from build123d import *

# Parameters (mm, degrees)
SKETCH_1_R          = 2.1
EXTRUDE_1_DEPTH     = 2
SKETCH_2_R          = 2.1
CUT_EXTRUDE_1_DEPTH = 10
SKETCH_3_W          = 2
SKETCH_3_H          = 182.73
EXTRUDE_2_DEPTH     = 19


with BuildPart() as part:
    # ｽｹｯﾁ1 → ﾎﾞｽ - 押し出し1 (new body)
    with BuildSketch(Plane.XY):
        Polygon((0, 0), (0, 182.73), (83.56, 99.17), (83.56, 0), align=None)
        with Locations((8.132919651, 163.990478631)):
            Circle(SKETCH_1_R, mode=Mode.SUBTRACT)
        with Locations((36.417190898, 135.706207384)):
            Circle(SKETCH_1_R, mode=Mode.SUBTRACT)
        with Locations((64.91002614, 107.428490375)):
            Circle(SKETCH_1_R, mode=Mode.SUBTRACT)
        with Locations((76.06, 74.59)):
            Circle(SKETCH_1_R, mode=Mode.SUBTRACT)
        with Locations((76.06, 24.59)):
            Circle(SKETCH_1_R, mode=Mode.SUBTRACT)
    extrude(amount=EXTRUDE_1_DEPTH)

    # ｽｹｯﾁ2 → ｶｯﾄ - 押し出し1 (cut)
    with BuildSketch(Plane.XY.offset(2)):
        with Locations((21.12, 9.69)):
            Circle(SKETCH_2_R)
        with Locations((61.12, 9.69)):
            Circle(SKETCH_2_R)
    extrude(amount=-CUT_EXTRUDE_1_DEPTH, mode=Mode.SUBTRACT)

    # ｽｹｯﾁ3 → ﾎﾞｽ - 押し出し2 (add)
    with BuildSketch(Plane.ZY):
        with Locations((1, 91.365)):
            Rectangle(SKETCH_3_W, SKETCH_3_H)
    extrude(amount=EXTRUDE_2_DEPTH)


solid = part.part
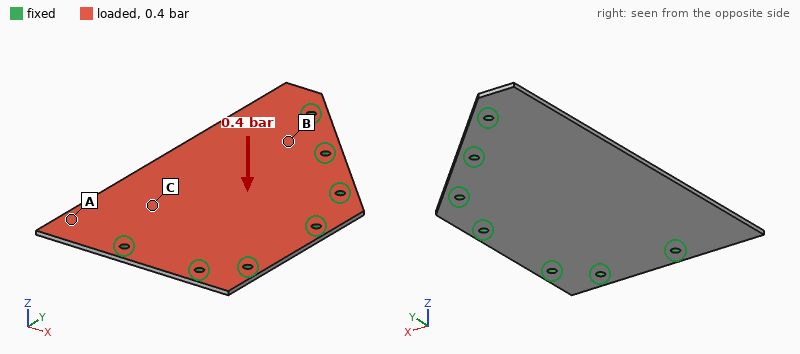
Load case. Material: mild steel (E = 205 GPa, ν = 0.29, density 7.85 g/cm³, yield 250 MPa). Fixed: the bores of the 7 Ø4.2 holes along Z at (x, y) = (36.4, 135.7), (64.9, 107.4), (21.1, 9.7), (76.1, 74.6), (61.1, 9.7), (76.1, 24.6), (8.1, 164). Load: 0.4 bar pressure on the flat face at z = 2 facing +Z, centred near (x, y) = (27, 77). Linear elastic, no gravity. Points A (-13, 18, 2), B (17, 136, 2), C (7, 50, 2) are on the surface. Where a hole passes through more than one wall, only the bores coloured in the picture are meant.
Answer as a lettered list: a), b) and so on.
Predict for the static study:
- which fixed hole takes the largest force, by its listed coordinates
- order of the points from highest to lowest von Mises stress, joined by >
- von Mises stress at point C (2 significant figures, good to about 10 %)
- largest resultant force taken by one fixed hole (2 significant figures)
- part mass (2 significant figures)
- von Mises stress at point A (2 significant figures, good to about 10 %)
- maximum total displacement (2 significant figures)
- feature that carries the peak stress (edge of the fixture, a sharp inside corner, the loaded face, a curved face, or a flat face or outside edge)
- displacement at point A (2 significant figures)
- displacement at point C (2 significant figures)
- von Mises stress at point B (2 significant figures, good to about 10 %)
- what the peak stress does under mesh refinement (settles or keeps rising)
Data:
a) (21.1, 9.7)
b) B > C > A
c) 30 MPa
d) 190 N
e) 240 g
f) 14 MPa
g) 0.48 mm
h) edge of the fixture
i) 0.19 mm
j) 0.25 mm
k) 44 MPa
l) keeps rising
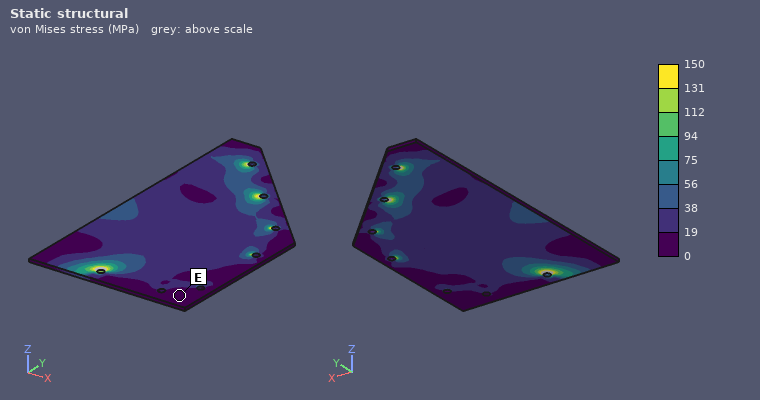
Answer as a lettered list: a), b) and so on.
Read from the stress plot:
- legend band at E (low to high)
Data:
a) 0 to 19 MPa
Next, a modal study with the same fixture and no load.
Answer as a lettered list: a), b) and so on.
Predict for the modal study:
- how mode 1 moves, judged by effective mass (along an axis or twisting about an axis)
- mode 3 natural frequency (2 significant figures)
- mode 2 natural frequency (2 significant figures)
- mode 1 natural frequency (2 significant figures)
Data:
a) along Z
b) 1300 Hz
c) 1100 Hz
d) 500 Hz
